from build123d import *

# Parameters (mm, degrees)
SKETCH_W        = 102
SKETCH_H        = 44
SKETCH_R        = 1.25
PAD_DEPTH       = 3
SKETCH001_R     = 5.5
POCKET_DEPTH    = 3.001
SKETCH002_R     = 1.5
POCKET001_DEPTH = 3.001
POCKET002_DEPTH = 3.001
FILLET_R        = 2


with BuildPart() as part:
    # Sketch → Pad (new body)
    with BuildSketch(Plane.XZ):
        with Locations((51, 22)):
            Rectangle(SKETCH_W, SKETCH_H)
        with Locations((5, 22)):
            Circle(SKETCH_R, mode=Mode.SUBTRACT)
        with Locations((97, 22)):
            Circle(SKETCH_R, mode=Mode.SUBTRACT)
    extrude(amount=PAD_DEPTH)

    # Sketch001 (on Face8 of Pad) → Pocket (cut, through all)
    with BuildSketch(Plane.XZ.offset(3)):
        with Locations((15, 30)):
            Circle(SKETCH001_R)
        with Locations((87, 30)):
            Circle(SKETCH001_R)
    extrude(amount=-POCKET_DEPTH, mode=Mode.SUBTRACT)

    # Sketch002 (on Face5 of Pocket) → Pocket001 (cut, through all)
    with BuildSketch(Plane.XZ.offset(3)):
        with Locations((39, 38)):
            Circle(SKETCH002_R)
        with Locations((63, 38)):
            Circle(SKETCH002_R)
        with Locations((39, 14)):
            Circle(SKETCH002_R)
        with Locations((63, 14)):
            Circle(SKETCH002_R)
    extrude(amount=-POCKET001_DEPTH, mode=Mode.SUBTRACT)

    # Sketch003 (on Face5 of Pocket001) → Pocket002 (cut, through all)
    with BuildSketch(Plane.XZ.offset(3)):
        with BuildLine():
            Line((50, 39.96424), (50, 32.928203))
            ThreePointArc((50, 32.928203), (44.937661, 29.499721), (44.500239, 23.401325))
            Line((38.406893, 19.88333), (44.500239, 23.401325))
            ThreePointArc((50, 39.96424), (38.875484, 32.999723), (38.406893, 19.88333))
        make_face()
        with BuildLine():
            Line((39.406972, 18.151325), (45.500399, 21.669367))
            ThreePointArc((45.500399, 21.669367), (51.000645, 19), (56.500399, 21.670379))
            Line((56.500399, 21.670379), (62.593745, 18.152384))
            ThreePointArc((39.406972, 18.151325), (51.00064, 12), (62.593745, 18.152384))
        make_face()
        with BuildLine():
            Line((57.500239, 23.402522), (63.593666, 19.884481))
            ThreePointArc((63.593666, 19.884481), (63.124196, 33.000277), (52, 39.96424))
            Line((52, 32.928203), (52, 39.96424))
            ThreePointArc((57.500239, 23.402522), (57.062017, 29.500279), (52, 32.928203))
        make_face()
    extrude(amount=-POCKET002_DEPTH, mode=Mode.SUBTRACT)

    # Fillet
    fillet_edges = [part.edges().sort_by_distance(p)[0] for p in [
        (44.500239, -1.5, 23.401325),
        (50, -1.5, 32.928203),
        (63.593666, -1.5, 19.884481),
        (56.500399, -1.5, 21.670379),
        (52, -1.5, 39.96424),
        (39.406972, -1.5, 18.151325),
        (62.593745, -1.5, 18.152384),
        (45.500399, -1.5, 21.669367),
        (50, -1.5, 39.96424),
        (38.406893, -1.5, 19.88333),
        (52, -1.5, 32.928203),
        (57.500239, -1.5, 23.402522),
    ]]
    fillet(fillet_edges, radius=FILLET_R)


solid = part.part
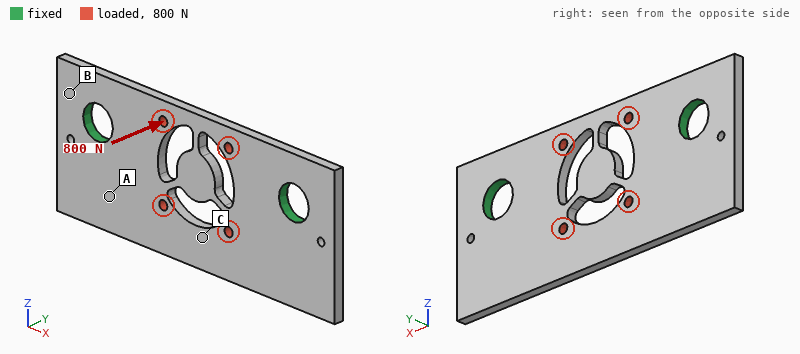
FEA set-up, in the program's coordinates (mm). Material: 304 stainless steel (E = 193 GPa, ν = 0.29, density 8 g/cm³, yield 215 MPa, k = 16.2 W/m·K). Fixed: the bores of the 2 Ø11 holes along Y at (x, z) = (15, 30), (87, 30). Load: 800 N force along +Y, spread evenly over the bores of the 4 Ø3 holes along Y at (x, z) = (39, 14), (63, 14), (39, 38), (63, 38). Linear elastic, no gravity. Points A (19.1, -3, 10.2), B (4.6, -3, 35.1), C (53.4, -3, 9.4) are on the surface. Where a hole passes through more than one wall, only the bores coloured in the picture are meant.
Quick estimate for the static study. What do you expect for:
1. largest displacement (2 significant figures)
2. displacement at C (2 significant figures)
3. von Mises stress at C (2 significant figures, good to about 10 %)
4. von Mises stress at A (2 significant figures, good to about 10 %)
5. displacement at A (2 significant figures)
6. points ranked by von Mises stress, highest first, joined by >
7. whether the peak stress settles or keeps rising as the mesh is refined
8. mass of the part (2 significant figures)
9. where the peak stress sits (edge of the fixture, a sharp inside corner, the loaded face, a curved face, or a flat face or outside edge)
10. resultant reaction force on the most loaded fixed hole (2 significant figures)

84 µm
77 µm
58 MPa
35 MPa
15 µm
C > A > B
keeps rising
92 g
edge of the fixture
400 N
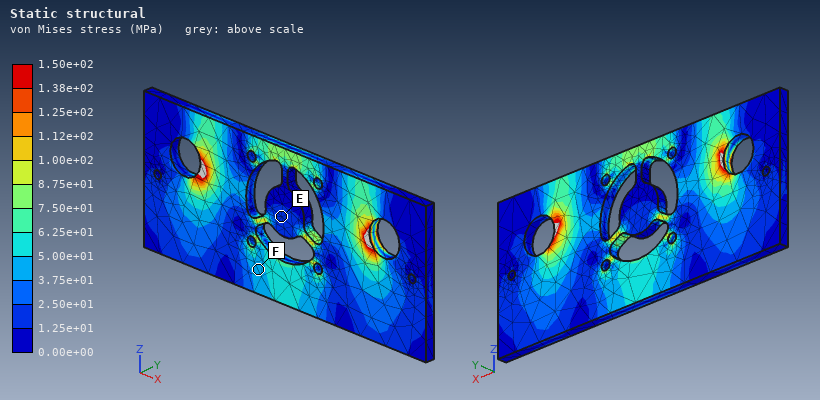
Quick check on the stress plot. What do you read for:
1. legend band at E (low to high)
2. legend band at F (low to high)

1.25e+01 to 2.50e+01 MPa
3.75e+01 to 5.00e+01 MPa
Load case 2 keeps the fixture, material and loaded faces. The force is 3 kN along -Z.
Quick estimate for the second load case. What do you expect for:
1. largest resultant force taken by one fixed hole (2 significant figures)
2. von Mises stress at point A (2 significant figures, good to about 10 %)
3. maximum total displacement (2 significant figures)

1.5 kN
9.9 MPa
8.9 µm
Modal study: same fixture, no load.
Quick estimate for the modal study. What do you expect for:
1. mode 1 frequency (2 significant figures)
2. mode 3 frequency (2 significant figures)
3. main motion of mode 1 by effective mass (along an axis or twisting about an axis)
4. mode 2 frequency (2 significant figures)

2300 Hz
3800 Hz
along Y
3700 Hz
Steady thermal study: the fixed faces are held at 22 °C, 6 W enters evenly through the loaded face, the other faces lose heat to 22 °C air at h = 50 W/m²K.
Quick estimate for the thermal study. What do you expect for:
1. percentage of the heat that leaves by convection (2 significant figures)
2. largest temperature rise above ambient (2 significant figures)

61 %
30 K
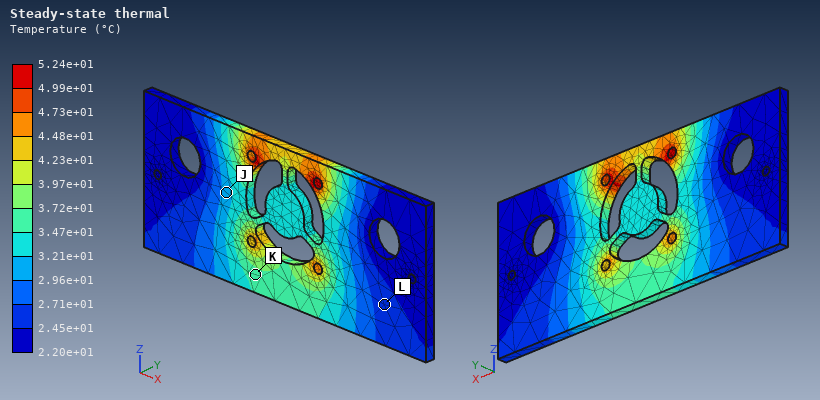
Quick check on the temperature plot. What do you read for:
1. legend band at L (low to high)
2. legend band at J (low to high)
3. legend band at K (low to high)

2.45e+01 to 2.71e+01 °C
2.96e+01 to 3.21e+01 °C
3.47e+01 to 3.72e+01 °C
